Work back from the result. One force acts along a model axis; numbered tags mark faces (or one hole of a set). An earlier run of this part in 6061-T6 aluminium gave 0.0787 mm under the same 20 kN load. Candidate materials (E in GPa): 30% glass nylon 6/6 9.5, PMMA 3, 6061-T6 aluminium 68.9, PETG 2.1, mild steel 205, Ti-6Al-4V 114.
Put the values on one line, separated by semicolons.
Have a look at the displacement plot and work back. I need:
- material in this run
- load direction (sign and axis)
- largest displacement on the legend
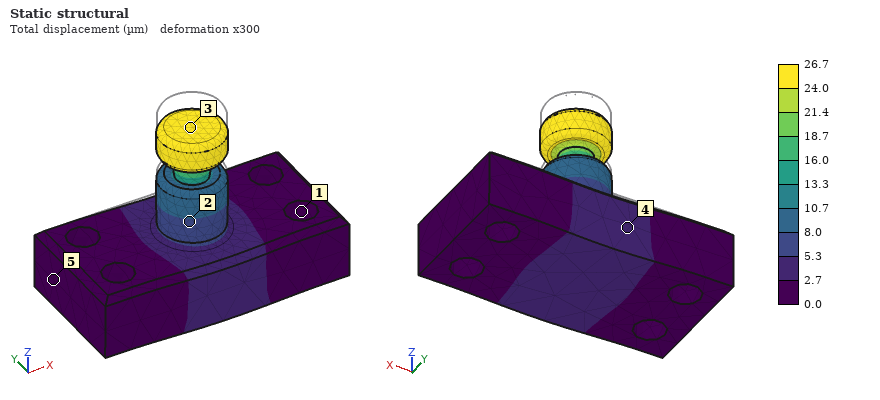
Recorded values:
mild steel; -Z; 26.7 µm
